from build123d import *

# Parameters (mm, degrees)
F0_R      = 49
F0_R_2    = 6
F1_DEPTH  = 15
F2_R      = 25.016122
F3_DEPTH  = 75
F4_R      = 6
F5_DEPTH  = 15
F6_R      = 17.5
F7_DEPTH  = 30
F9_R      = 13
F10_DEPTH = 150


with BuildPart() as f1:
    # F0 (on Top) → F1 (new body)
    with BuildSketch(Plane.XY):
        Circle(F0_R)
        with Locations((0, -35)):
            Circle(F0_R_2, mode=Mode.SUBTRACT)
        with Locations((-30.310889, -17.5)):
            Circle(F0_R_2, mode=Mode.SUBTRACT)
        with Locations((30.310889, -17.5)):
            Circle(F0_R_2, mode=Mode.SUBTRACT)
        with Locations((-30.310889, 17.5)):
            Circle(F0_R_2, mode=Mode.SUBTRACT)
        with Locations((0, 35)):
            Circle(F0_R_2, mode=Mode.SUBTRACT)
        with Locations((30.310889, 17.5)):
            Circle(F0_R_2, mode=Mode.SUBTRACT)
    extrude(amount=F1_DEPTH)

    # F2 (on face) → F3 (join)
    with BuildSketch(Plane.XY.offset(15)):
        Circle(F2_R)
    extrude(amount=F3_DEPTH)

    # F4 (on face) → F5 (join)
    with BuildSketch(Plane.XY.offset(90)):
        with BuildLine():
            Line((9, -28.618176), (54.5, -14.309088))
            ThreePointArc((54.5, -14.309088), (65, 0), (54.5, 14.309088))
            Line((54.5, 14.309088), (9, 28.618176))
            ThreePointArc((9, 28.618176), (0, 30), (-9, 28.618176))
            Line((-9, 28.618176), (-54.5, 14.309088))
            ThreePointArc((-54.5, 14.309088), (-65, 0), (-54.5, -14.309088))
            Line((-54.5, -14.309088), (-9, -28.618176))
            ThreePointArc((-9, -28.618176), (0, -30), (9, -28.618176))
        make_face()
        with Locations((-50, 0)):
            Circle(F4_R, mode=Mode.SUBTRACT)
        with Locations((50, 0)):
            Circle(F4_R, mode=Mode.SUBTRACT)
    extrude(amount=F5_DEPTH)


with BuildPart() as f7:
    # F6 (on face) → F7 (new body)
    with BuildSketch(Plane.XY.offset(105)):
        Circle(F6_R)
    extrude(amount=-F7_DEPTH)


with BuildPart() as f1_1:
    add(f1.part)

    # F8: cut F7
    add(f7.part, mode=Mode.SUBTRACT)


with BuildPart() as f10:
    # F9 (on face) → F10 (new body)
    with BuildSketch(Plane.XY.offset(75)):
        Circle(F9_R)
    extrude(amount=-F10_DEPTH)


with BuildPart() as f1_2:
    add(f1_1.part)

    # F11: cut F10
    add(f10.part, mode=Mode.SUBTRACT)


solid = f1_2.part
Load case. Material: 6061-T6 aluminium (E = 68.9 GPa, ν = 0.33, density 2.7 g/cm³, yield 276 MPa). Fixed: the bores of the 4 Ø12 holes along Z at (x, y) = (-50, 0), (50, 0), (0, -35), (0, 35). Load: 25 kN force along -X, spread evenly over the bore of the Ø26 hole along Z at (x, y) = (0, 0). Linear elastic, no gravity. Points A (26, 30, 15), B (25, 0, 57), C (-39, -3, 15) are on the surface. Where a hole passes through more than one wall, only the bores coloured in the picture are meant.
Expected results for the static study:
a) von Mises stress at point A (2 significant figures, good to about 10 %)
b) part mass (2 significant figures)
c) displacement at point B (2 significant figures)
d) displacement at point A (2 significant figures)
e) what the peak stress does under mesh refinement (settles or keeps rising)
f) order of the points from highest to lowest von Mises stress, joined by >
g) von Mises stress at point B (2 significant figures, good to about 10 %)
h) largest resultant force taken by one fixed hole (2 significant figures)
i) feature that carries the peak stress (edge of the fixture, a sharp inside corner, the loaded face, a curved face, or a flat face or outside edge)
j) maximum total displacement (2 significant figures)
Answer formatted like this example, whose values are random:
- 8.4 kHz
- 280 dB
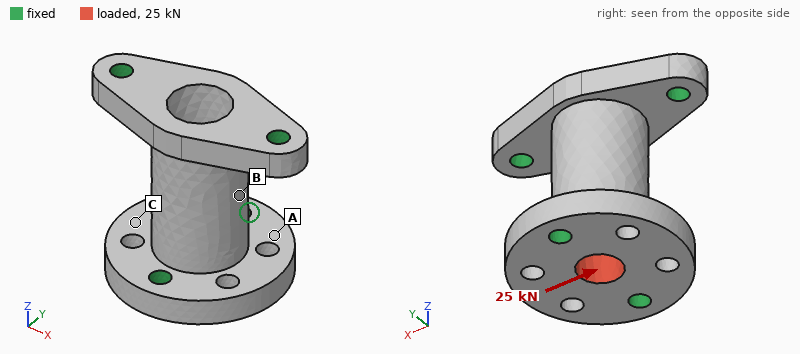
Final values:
- 10.0 MPa
- 700 g
- 24 µm
- 8.7 µm
- keeps rising
- B > A > C
- 20 MPa
- 8.0 kN
- edge of the fixture
- 26 µm
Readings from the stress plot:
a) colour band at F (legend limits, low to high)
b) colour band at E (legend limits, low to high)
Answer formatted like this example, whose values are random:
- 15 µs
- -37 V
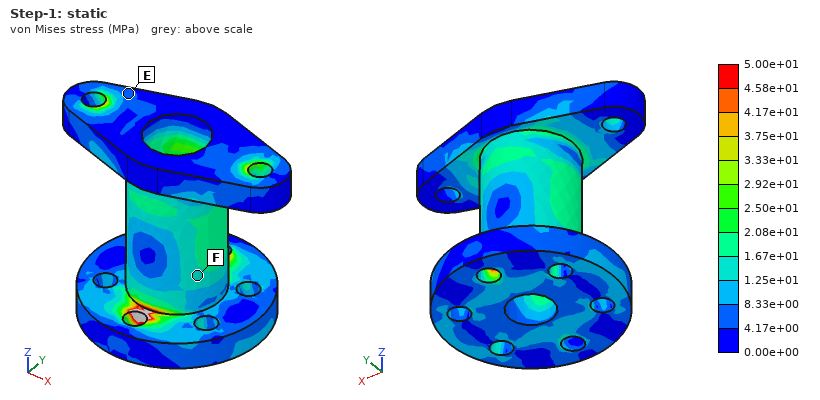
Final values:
- 1.25e+01 to 1.67e+01 MPa
- 4.17e+00 to 8.33e+00 MPa
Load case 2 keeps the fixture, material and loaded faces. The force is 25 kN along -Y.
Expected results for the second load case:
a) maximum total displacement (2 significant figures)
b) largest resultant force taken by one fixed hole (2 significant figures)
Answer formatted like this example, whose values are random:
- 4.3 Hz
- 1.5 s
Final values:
- 25 µm
- 10 kN
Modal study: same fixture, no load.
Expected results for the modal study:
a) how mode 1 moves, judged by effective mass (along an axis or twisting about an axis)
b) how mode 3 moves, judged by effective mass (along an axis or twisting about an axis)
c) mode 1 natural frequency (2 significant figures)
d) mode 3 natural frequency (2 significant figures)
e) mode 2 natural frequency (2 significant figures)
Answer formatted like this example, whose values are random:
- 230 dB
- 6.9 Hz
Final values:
- along Z
- along Y
- 7000 Hz
- 8800 Hz
- 7600 Hz
